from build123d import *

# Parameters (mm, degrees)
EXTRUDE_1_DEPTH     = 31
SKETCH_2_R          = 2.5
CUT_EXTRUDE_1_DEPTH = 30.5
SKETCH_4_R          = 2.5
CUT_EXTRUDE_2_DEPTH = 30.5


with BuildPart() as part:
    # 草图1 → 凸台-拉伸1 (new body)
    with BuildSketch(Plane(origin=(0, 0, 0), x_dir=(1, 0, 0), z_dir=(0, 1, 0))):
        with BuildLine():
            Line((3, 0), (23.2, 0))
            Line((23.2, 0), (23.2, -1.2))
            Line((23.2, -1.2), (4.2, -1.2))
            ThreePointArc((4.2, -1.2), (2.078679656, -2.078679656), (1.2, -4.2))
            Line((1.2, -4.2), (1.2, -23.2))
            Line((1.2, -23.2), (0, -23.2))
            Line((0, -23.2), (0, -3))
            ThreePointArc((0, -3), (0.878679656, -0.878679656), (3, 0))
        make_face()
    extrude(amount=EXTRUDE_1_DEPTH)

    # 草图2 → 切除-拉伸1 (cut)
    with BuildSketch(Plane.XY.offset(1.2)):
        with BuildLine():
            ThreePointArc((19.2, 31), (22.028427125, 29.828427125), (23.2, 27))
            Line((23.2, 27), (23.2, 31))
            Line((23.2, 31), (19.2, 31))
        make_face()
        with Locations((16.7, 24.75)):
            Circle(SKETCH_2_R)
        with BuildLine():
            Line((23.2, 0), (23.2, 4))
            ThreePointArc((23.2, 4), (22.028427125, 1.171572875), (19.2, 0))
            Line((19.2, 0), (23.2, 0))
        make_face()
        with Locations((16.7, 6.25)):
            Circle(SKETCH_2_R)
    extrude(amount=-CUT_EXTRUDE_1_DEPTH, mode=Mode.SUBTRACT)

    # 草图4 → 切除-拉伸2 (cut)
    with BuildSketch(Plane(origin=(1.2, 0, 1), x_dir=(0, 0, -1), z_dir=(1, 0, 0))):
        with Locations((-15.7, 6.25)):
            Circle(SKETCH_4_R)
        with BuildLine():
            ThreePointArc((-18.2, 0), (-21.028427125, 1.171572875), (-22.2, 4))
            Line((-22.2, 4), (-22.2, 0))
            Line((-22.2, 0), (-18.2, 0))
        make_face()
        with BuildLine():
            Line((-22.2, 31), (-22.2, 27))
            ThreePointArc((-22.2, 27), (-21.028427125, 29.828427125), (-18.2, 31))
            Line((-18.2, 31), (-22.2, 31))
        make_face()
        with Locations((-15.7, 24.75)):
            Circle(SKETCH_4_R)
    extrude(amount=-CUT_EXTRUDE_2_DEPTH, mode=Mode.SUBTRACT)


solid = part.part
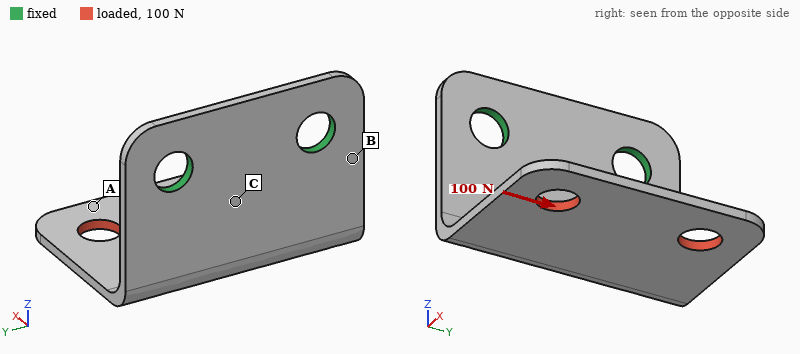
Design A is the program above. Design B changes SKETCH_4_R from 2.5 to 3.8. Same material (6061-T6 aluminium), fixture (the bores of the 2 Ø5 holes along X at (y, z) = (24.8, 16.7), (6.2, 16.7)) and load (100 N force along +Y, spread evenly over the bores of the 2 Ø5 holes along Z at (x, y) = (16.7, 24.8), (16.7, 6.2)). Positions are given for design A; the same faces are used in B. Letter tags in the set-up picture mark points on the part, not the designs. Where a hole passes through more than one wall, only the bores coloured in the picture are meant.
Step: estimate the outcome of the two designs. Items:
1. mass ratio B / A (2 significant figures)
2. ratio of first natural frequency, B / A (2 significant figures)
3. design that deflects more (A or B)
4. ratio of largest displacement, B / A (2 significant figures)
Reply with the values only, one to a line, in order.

0.96
1.1
A
0.81
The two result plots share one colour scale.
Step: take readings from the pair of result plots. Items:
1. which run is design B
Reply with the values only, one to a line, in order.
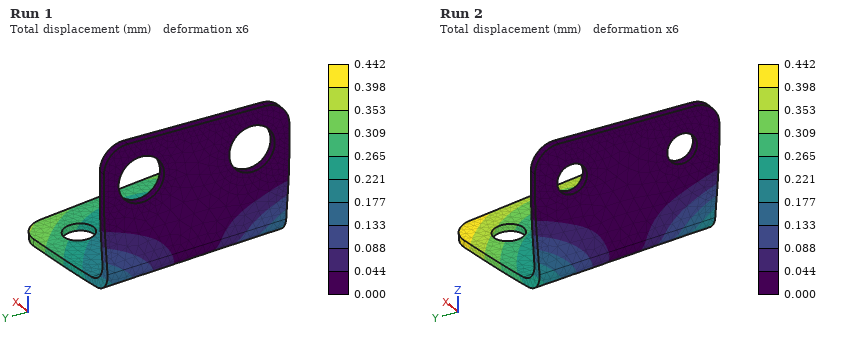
Run 1
